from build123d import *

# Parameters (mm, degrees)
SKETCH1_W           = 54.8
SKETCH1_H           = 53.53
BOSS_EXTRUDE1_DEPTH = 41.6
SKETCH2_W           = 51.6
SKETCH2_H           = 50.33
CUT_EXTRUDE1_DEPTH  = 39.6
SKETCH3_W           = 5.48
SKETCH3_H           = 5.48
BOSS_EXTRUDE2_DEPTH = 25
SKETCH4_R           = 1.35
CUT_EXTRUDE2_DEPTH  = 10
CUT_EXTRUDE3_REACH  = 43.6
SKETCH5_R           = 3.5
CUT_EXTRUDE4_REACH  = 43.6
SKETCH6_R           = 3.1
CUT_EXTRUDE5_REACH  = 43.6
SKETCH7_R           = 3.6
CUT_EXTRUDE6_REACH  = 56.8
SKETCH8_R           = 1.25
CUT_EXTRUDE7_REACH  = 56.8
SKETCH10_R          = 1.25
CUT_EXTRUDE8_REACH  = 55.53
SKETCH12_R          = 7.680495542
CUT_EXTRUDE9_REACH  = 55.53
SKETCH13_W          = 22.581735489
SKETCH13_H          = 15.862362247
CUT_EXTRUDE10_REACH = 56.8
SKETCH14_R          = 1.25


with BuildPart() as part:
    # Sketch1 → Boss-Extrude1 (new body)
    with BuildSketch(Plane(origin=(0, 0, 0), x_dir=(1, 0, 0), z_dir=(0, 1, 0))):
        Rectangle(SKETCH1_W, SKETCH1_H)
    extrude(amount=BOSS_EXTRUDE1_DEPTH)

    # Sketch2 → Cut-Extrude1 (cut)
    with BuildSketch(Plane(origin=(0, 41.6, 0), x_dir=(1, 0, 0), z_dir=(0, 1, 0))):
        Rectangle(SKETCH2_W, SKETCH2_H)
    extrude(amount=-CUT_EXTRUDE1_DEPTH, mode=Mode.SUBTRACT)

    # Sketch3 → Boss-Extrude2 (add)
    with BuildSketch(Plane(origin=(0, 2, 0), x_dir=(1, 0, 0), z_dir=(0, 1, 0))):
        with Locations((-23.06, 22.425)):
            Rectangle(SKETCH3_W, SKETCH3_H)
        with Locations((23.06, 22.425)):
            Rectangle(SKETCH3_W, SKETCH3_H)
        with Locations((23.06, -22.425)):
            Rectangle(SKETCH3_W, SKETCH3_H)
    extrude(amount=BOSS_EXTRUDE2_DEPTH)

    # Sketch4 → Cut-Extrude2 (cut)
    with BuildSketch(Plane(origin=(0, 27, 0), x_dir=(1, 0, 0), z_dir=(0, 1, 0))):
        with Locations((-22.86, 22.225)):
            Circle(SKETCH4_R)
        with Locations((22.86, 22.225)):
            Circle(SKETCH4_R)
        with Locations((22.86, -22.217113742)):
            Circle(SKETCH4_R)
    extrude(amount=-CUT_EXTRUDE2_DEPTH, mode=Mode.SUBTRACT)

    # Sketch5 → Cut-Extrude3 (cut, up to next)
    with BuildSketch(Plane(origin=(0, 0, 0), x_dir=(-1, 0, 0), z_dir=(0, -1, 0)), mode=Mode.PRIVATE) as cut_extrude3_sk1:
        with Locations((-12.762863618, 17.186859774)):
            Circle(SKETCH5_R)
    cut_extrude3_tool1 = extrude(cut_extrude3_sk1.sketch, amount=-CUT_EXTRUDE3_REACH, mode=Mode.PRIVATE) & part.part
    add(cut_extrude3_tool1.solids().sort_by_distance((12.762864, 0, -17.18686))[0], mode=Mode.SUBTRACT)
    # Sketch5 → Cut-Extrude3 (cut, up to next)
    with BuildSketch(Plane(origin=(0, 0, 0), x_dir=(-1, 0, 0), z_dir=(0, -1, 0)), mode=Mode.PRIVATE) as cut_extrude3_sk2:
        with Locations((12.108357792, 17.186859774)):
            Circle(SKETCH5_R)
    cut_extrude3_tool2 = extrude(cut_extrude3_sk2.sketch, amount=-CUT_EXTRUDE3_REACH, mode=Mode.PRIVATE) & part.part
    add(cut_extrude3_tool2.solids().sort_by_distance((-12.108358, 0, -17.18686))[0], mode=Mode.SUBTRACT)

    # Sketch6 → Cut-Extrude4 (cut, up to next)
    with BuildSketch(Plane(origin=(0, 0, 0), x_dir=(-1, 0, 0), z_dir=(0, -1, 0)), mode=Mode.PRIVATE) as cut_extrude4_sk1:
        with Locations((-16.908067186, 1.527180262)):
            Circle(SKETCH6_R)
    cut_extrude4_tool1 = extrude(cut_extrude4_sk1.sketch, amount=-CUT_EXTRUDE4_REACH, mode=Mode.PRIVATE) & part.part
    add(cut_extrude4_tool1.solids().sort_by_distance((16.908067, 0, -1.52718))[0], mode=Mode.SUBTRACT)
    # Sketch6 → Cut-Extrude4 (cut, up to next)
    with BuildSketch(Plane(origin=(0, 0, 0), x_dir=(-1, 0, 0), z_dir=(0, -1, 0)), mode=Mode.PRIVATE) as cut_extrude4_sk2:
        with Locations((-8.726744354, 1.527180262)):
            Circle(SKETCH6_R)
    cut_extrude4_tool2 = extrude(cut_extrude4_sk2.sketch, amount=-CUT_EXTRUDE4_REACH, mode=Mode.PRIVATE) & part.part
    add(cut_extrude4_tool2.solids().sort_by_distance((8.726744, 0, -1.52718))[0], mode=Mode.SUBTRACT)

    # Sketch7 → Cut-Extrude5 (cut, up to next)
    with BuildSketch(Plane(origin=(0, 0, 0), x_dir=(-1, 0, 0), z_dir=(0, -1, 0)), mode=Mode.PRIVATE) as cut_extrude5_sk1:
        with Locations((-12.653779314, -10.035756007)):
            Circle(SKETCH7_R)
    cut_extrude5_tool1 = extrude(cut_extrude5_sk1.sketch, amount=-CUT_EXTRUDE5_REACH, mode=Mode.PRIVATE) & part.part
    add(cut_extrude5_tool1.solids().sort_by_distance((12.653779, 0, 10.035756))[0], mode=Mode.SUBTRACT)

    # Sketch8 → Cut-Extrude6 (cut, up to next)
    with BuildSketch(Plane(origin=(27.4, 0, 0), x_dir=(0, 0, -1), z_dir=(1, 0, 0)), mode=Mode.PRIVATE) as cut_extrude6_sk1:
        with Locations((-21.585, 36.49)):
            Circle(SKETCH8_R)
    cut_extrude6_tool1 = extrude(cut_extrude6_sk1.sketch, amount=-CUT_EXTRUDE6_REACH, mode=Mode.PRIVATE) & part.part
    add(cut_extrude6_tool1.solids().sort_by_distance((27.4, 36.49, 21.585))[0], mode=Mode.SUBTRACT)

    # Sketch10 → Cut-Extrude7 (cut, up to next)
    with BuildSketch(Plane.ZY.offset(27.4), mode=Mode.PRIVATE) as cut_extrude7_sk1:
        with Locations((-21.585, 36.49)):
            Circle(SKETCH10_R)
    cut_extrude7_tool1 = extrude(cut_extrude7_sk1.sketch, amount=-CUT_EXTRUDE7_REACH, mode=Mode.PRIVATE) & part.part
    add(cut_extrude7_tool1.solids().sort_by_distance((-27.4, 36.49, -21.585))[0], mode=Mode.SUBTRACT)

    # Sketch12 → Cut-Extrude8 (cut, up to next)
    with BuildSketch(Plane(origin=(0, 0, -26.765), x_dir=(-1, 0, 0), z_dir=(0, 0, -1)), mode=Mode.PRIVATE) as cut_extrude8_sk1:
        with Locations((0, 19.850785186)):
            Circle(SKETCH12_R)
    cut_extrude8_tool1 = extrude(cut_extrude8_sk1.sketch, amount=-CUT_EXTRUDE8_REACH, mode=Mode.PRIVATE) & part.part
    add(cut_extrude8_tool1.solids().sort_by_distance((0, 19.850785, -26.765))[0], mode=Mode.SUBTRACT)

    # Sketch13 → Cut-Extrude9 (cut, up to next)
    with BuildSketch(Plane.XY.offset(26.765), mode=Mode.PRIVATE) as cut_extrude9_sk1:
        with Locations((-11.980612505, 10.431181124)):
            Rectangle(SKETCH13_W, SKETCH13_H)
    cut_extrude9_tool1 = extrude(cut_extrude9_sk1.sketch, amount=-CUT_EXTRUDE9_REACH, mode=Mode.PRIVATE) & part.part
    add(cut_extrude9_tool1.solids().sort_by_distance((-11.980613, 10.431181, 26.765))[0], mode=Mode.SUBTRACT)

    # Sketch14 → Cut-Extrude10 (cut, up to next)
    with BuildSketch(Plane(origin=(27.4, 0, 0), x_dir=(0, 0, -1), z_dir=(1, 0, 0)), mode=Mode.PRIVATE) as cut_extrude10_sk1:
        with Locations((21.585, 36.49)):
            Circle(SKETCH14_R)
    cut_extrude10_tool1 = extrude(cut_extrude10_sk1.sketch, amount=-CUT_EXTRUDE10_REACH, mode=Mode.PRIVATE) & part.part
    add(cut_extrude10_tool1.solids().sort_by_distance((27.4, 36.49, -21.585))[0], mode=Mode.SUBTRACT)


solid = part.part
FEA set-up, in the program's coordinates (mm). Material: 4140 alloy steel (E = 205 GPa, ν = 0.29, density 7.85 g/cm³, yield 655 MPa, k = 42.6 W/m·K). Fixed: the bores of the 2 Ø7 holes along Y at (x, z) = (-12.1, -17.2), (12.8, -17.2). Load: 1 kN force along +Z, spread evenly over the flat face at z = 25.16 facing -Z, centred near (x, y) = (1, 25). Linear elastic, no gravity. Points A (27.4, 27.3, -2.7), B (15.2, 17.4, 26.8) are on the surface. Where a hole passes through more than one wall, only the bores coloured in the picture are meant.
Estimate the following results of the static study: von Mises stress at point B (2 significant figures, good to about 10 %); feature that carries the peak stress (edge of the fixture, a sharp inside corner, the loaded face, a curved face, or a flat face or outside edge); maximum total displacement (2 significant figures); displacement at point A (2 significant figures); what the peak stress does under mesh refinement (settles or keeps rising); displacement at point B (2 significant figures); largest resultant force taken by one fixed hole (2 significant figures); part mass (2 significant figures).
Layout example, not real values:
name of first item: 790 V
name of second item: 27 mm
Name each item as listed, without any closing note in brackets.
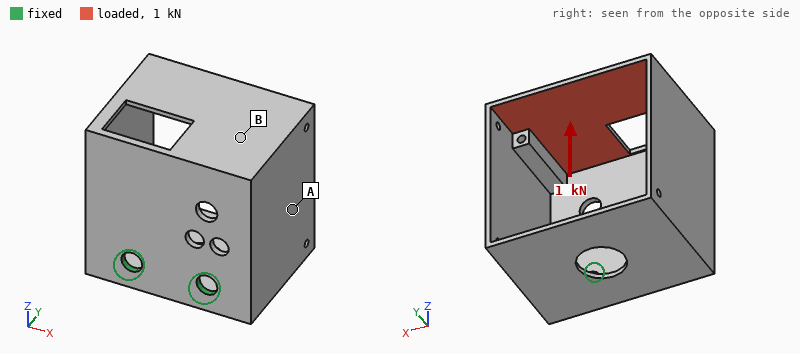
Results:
von Mises stress at point B: 99 MPa
feature that carries the peak stress: edge of the fixture
maximum total displacement: 0.66 mm
displacement at point A: 0.23 mm
what the peak stress does under mesh refinement: keeps rising
displacement at point B: 0.38 mm
largest resultant force taken by one fixed hole: 500 N
part mass: 160 g
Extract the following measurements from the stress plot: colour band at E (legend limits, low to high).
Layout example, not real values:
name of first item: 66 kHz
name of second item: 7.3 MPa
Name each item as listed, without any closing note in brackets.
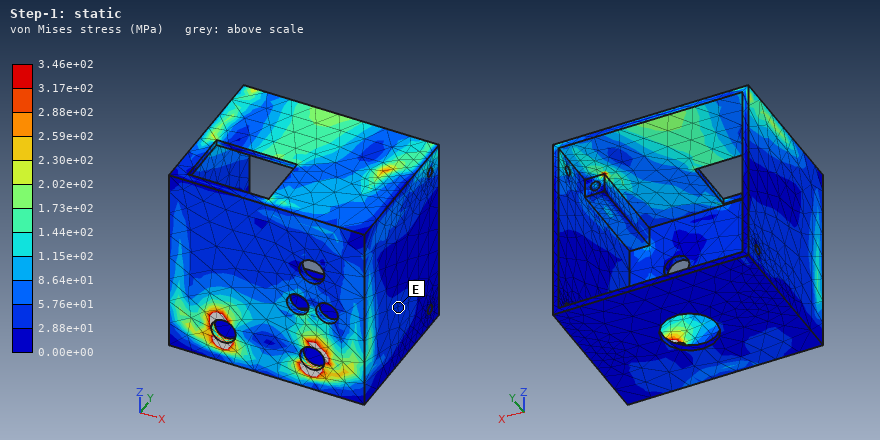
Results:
colour band at E: 2.88e+01 to 5.76e+01 MPa
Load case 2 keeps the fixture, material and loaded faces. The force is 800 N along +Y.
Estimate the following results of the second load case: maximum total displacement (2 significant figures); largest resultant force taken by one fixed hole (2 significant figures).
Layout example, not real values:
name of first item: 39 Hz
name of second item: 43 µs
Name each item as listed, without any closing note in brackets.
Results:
maximum total displacement: 0.69 mm
largest resultant force taken by one fixed hole: 430 N
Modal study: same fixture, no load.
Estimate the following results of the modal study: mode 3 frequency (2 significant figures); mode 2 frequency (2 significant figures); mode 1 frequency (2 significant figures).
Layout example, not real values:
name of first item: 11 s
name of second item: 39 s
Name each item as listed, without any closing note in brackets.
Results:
mode 3 frequency: 2500 Hz
mode 2 frequency: 950 Hz
mode 1 frequency: 690 Hz
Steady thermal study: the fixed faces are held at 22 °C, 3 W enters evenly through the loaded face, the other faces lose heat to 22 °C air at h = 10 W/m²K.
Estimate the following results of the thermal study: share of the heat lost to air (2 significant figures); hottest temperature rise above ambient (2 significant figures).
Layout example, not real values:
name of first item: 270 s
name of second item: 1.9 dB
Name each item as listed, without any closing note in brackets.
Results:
share of the heat lost to air: 45 %
hottest temperature rise above ambient: 21 K
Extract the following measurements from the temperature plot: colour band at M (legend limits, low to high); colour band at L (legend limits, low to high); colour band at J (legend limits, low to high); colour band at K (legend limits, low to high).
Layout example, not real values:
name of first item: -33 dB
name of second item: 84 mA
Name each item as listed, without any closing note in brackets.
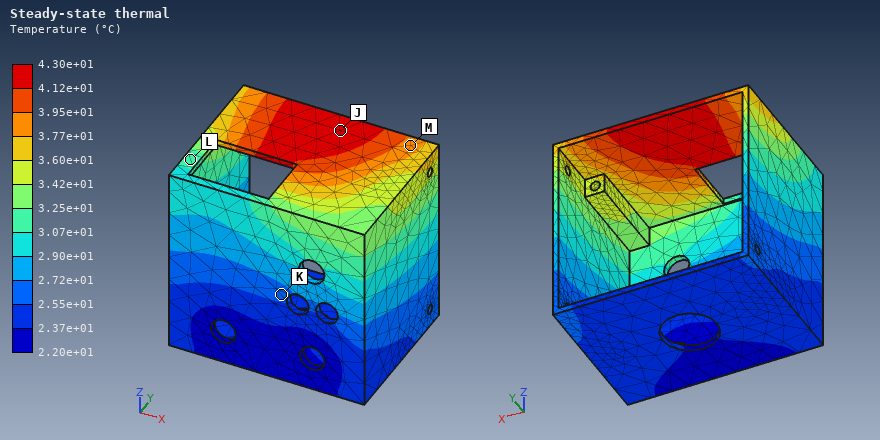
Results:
colour band at M: 3.77e+01 to 3.95e+01 °C
colour band at L: 3.07e+01 to 3.25e+01 °C
colour band at J: 4.12e+01 to 4.30e+01 °C
colour band at K: 2.55e+01 to 2.72e+01 °C
